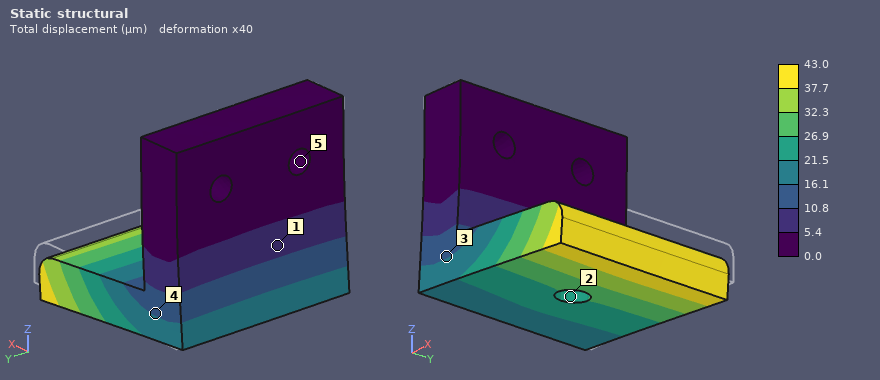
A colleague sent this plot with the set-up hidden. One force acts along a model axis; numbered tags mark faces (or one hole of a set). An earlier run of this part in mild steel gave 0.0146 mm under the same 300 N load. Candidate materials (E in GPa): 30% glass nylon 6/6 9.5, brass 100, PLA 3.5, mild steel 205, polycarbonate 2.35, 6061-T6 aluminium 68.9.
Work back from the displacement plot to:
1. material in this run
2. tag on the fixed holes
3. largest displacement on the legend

6061-T6 aluminium
5
43.0 µm
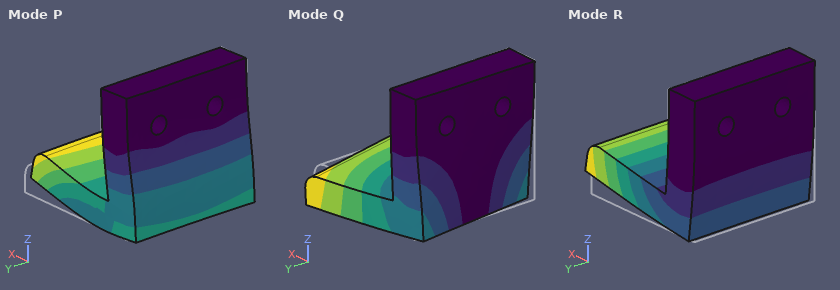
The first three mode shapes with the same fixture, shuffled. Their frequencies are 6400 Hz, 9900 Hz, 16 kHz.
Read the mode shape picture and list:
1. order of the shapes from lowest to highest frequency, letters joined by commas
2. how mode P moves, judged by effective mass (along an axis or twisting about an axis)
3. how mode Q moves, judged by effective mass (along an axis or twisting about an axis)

R, Q, P
along X
along Y
